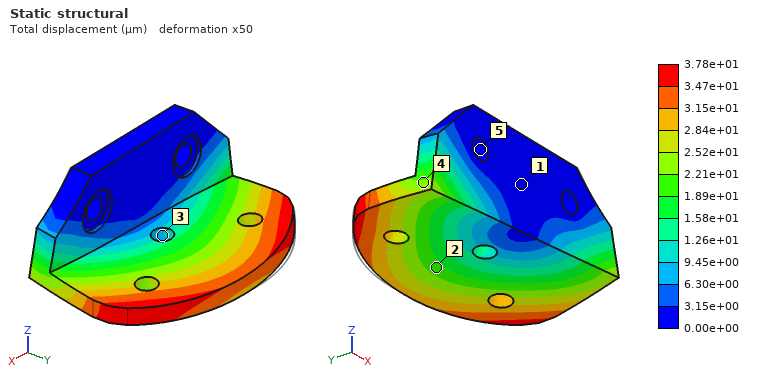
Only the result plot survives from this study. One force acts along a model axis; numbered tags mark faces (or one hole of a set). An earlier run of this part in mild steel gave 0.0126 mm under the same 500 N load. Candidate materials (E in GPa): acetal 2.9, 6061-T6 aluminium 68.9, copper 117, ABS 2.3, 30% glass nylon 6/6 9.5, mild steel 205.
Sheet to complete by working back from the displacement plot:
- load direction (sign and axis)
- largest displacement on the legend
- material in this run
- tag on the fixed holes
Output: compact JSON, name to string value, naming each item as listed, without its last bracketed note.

{"load direction": "+X", "largest displacement on the legend": "3.78e+01 µm", "material in this run": "6061-T6 aluminium", "tag on the fixed holes": "5"}
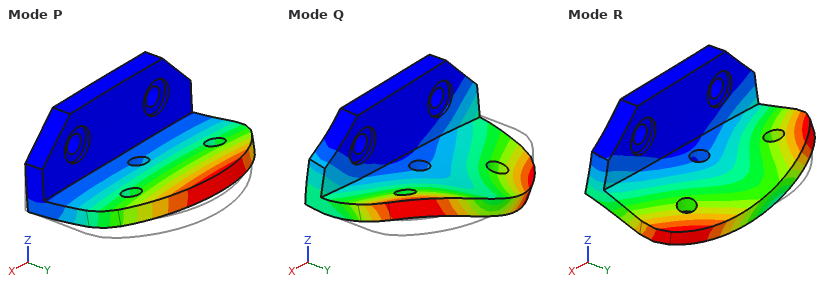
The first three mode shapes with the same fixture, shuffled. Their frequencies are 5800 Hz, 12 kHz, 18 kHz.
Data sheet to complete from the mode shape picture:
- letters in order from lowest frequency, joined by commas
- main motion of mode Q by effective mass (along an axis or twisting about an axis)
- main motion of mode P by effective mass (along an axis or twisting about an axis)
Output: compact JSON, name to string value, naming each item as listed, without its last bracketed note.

{"letters in order from lowest frequency, joined by commas": "P, R, Q", "main motion of mode Q by effective mass": "along X", "main motion of mode P by effective mass": "along Z"}
